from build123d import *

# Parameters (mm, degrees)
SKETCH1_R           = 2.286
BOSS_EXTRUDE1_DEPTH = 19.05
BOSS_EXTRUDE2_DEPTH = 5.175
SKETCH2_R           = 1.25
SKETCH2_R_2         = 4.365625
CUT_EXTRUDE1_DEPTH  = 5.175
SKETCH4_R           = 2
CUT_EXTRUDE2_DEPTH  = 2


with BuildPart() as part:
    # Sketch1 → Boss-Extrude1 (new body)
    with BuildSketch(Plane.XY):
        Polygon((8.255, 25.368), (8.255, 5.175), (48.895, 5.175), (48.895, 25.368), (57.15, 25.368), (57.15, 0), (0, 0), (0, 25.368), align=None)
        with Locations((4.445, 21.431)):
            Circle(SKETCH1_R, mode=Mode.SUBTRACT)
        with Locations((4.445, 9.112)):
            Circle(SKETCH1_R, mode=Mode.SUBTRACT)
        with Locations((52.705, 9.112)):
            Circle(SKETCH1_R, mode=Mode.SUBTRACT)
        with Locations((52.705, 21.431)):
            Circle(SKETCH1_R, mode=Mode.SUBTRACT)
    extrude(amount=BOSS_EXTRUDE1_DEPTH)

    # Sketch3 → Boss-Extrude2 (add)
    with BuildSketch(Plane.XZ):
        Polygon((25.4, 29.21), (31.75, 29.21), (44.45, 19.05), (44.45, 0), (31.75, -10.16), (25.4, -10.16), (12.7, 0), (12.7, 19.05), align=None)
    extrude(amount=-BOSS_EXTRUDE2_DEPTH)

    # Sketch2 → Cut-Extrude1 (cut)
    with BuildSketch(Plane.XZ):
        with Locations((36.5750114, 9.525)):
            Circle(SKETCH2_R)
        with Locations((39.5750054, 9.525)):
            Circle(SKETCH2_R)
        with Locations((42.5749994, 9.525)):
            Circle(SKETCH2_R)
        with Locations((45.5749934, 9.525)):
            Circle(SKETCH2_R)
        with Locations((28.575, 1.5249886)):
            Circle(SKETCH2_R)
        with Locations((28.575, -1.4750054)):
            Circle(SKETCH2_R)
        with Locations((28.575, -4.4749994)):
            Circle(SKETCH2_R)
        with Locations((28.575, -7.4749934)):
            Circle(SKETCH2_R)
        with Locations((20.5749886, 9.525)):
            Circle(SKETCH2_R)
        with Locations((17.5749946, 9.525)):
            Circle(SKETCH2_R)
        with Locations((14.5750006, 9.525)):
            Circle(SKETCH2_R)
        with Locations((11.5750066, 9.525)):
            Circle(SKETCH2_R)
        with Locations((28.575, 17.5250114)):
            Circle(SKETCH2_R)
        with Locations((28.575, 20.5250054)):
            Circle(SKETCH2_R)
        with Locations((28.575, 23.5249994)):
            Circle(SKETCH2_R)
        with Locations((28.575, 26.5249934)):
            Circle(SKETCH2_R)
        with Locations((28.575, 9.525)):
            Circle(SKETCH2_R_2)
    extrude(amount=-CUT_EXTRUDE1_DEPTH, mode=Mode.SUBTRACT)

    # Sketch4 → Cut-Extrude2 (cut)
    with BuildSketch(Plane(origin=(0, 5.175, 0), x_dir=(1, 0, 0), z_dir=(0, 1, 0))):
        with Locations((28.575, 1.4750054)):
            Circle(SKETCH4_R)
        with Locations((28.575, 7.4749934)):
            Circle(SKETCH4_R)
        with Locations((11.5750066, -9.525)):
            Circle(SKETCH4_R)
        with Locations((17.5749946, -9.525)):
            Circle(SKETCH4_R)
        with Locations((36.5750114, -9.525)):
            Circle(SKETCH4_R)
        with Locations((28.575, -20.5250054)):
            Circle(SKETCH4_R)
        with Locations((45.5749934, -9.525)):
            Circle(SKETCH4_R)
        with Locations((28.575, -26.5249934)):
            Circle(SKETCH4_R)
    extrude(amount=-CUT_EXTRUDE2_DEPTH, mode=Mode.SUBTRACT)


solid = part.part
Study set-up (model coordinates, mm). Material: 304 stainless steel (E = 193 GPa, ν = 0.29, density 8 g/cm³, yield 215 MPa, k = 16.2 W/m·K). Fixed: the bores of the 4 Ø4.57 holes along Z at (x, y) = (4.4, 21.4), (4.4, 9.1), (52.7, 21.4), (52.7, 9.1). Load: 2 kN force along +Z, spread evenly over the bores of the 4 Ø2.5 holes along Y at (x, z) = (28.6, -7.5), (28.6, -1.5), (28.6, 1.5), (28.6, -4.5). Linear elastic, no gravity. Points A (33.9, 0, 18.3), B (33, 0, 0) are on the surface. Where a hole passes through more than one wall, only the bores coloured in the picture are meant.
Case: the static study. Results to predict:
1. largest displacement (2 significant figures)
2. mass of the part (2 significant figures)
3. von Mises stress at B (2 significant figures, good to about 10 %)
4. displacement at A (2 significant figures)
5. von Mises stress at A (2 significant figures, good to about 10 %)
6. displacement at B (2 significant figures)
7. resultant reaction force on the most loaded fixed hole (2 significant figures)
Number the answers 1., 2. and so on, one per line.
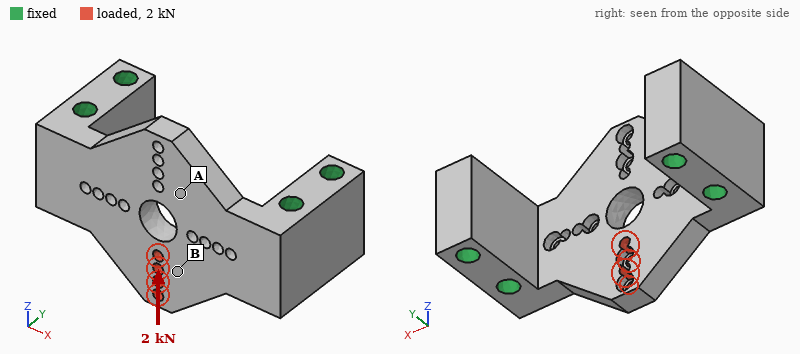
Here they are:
1. 9.2 µm
2. 95 g
3. 31 MPa
4. 4.1 µm
5. 13 MPa
6. 6.6 µm
7. 1.0 kN
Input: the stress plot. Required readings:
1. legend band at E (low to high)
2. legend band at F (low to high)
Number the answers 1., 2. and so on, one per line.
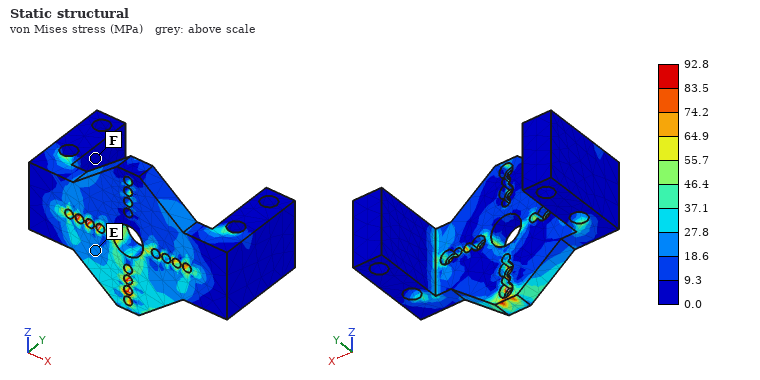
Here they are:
1. 18.6 to 27.8 MPa
2. 0.0 to 9.3 MPa
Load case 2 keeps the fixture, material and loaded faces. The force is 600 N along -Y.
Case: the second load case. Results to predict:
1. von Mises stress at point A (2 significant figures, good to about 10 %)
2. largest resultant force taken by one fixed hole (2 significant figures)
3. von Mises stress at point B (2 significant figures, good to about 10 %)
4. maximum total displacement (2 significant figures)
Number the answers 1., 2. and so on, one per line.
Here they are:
1. 12 MPa
2. 460 N
3. 36 MPa
4. 33 µm
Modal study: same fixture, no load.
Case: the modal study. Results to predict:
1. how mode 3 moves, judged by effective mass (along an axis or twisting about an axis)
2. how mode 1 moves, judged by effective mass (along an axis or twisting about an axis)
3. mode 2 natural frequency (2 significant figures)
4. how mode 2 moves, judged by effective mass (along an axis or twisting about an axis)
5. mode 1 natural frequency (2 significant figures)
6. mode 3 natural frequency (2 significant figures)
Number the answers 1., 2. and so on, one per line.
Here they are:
1. along Z
2. along Y
3. 8700 Hz
4. twisting about X
5. 8300 Hz
6. 19 kHz
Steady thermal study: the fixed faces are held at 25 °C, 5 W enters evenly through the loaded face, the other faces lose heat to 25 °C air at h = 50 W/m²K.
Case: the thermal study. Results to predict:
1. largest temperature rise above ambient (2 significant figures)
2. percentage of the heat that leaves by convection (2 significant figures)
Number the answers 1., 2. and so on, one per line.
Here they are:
1. 47 K
2. 48 %
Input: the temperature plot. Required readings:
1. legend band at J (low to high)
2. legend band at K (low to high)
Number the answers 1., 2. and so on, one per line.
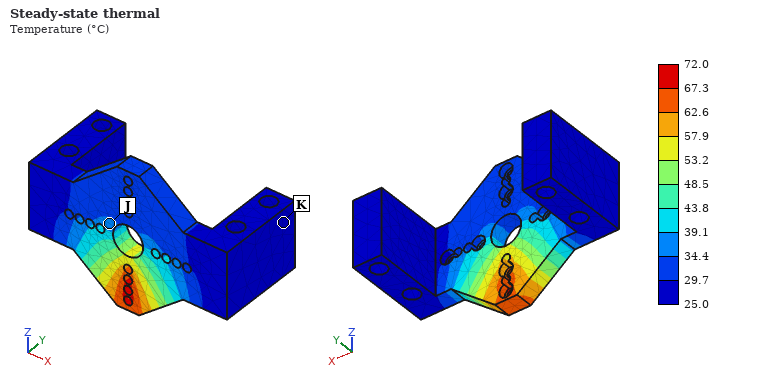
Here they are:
1. 34.4 to 39.1 °C
2. 25.0 to 29.7 °C
